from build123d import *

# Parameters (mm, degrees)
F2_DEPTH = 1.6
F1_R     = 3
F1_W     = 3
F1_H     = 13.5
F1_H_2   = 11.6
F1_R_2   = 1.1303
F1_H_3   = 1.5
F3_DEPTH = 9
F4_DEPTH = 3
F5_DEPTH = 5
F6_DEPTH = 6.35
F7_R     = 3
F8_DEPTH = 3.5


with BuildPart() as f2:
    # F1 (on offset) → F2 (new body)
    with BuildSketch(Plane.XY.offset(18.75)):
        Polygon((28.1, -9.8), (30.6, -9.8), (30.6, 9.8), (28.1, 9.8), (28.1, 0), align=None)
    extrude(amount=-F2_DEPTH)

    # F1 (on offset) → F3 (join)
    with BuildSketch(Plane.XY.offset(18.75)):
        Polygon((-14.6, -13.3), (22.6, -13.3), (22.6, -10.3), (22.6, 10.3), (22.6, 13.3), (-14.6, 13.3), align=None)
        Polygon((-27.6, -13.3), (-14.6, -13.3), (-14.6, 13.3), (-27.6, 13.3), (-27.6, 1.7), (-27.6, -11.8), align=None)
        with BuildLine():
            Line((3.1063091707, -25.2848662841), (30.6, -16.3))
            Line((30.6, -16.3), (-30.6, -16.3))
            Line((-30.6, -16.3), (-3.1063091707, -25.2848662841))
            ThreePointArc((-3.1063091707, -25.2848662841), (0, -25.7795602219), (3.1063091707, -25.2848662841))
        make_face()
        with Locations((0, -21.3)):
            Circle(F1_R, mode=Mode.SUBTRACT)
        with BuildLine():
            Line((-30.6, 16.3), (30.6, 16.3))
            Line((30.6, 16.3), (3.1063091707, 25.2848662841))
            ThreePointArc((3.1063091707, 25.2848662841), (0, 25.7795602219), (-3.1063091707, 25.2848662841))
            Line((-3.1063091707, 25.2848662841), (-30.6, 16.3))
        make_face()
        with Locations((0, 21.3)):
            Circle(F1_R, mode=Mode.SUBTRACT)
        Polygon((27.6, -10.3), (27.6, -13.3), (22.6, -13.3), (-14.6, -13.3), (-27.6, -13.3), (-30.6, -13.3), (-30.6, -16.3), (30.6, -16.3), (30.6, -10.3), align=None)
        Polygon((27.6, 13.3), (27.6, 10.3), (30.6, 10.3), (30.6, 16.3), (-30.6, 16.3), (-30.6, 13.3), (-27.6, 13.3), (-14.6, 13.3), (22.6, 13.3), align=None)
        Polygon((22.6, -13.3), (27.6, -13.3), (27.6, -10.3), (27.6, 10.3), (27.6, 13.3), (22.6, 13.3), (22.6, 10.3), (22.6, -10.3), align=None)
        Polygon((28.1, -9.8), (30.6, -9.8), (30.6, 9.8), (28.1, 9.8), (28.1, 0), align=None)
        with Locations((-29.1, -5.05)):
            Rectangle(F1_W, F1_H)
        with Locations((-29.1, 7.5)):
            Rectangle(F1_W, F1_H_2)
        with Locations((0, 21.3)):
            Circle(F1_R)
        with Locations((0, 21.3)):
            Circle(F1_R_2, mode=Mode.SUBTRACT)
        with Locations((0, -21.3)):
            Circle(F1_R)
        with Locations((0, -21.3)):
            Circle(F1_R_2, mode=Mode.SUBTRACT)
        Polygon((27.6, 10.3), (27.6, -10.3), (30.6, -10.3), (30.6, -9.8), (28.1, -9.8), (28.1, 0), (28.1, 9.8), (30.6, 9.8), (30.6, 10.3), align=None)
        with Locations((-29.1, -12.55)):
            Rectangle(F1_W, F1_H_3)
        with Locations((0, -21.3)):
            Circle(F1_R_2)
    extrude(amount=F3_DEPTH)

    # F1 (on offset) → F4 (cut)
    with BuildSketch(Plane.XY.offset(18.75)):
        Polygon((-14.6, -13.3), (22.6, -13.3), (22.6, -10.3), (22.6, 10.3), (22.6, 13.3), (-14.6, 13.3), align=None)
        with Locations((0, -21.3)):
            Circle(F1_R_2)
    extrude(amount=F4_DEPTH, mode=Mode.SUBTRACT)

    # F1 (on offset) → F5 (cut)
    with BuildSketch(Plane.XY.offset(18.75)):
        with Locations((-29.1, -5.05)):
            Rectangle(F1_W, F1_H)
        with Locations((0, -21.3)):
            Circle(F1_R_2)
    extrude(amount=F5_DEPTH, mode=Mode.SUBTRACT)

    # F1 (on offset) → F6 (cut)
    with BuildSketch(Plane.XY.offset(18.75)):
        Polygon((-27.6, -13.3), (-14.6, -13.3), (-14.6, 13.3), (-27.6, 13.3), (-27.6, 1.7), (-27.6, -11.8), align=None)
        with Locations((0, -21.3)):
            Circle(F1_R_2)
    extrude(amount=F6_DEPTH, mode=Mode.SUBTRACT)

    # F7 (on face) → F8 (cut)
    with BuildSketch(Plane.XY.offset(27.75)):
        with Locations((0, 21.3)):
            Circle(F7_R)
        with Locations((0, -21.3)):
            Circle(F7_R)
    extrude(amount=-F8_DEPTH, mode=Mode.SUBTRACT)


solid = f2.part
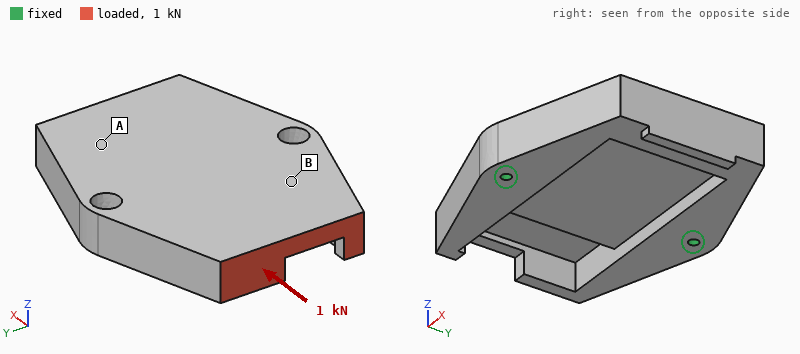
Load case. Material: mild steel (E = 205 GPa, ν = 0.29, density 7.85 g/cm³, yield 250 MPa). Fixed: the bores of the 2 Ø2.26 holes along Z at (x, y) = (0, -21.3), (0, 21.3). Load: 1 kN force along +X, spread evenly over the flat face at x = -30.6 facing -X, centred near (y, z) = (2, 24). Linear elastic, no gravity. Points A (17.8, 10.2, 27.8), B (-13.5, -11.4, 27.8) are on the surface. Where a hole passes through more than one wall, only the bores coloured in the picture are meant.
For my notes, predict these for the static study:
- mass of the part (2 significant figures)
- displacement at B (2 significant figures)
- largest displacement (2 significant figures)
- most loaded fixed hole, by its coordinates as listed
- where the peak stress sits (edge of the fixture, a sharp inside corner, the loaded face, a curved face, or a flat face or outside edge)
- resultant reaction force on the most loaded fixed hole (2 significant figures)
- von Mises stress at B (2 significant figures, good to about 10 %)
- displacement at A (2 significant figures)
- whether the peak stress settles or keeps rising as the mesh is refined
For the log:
140 g
2.4 µm
7.8 µm
(0, 21.3)
edge of the fixture
540 N
6.7 MPa
2.1 µm
keeps rising
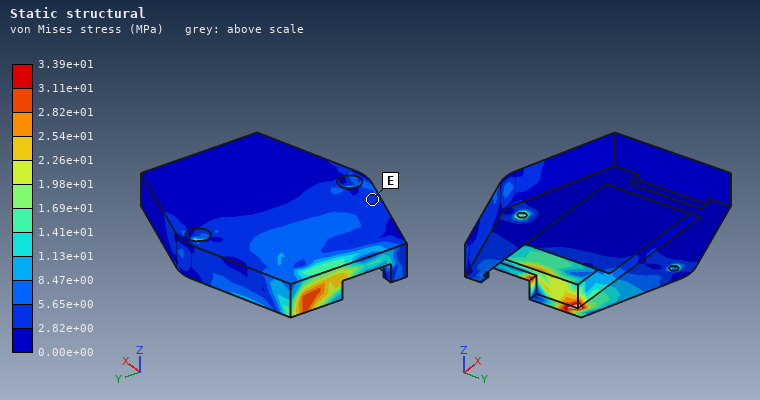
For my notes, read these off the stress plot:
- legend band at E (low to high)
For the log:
2.82e+00 to 5.65e+00 MPa
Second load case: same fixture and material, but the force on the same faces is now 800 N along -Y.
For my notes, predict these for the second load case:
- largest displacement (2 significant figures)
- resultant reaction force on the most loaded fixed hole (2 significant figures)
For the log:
9.4 µm
710 N
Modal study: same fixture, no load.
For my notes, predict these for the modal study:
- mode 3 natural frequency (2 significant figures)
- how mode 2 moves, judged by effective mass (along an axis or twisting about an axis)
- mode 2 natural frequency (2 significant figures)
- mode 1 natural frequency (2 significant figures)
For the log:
9000 Hz
along Z
6700 Hz
3400 Hz
